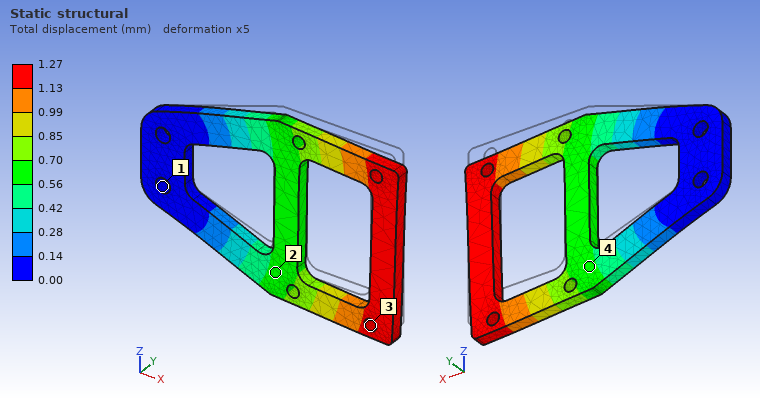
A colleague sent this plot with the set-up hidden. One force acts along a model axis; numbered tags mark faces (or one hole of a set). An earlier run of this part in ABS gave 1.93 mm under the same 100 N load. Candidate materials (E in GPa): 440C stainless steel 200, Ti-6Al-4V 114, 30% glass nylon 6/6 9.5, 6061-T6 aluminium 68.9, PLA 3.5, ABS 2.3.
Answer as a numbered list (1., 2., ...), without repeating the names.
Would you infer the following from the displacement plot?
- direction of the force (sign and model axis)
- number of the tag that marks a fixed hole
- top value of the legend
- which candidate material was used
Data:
1. -Z
2. 1
3. 1.27 mm
4. PLA
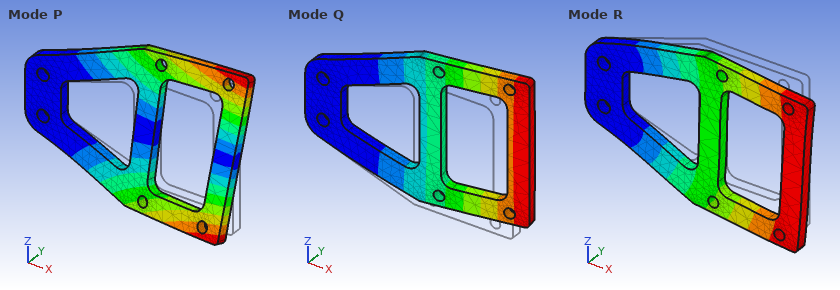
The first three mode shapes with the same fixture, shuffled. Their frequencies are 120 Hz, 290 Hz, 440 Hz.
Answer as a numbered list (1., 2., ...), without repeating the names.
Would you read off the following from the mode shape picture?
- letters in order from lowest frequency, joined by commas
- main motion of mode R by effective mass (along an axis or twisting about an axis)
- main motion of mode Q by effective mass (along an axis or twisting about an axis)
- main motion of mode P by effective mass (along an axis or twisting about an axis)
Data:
1. Q, P, R
2. along Z
3. along Y
4. twisting about X
